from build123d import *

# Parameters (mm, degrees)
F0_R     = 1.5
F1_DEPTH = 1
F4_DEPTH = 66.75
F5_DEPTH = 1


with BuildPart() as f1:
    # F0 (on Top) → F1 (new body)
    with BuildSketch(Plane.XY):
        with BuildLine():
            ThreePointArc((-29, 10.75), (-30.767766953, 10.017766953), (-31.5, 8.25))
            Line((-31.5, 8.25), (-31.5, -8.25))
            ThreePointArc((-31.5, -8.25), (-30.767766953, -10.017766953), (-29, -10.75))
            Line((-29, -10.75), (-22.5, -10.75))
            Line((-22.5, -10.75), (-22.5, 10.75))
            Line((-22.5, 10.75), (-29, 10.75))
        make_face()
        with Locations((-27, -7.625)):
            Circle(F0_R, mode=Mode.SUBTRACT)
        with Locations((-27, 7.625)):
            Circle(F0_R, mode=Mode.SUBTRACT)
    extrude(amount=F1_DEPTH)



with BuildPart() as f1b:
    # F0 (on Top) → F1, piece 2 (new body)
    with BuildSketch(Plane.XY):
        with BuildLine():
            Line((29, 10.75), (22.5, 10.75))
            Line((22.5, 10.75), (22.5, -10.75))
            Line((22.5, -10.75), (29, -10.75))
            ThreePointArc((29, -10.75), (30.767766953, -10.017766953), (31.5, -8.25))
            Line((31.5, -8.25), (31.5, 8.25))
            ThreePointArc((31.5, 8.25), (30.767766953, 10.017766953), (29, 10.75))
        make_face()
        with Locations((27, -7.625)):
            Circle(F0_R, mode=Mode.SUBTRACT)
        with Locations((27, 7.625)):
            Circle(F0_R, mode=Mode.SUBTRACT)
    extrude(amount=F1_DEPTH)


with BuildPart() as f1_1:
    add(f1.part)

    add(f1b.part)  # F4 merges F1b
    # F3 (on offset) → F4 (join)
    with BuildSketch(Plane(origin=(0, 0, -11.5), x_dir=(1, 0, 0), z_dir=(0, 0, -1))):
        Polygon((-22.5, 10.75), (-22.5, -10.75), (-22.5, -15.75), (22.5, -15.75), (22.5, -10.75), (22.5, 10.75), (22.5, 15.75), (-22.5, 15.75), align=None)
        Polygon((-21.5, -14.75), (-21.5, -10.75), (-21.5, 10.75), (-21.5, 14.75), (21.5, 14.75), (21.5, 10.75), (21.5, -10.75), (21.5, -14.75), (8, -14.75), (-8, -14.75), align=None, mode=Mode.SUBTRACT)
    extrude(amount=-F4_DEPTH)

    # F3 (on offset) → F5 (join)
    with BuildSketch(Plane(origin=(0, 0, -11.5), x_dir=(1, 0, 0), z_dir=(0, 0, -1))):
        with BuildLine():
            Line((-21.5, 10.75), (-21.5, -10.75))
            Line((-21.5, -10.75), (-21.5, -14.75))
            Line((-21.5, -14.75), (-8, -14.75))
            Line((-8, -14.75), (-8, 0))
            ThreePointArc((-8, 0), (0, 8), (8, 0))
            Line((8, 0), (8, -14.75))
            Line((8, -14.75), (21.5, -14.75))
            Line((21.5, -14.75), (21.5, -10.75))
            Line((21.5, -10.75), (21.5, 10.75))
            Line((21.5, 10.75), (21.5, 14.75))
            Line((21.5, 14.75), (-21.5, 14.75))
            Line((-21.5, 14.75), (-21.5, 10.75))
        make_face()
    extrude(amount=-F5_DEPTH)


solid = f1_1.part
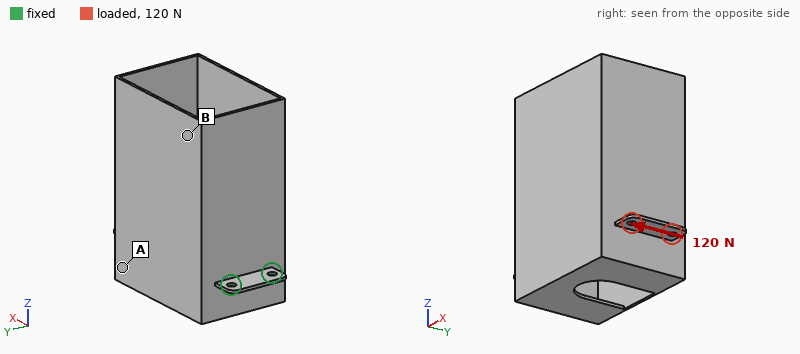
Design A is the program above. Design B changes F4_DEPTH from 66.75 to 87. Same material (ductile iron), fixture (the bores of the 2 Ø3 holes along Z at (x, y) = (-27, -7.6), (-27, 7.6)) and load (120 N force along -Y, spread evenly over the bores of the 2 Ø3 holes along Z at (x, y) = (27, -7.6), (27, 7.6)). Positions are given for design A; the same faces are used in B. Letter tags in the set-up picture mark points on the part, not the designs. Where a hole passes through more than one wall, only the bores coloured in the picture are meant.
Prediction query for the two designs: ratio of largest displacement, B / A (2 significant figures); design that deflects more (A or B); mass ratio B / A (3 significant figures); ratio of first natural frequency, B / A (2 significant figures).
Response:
0.79
A
1.27
0.74
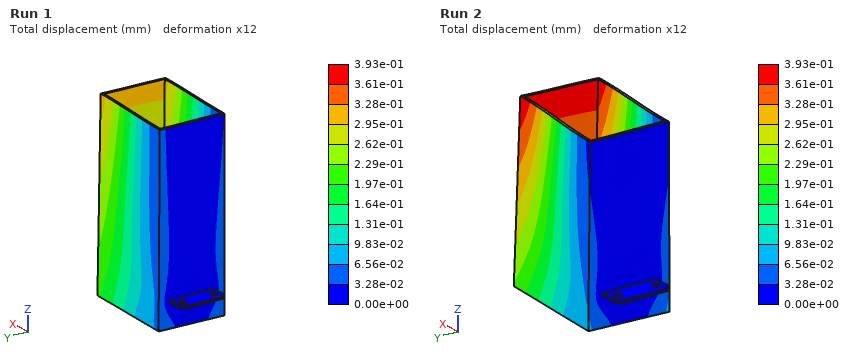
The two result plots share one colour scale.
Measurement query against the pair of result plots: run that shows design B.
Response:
Run 1
